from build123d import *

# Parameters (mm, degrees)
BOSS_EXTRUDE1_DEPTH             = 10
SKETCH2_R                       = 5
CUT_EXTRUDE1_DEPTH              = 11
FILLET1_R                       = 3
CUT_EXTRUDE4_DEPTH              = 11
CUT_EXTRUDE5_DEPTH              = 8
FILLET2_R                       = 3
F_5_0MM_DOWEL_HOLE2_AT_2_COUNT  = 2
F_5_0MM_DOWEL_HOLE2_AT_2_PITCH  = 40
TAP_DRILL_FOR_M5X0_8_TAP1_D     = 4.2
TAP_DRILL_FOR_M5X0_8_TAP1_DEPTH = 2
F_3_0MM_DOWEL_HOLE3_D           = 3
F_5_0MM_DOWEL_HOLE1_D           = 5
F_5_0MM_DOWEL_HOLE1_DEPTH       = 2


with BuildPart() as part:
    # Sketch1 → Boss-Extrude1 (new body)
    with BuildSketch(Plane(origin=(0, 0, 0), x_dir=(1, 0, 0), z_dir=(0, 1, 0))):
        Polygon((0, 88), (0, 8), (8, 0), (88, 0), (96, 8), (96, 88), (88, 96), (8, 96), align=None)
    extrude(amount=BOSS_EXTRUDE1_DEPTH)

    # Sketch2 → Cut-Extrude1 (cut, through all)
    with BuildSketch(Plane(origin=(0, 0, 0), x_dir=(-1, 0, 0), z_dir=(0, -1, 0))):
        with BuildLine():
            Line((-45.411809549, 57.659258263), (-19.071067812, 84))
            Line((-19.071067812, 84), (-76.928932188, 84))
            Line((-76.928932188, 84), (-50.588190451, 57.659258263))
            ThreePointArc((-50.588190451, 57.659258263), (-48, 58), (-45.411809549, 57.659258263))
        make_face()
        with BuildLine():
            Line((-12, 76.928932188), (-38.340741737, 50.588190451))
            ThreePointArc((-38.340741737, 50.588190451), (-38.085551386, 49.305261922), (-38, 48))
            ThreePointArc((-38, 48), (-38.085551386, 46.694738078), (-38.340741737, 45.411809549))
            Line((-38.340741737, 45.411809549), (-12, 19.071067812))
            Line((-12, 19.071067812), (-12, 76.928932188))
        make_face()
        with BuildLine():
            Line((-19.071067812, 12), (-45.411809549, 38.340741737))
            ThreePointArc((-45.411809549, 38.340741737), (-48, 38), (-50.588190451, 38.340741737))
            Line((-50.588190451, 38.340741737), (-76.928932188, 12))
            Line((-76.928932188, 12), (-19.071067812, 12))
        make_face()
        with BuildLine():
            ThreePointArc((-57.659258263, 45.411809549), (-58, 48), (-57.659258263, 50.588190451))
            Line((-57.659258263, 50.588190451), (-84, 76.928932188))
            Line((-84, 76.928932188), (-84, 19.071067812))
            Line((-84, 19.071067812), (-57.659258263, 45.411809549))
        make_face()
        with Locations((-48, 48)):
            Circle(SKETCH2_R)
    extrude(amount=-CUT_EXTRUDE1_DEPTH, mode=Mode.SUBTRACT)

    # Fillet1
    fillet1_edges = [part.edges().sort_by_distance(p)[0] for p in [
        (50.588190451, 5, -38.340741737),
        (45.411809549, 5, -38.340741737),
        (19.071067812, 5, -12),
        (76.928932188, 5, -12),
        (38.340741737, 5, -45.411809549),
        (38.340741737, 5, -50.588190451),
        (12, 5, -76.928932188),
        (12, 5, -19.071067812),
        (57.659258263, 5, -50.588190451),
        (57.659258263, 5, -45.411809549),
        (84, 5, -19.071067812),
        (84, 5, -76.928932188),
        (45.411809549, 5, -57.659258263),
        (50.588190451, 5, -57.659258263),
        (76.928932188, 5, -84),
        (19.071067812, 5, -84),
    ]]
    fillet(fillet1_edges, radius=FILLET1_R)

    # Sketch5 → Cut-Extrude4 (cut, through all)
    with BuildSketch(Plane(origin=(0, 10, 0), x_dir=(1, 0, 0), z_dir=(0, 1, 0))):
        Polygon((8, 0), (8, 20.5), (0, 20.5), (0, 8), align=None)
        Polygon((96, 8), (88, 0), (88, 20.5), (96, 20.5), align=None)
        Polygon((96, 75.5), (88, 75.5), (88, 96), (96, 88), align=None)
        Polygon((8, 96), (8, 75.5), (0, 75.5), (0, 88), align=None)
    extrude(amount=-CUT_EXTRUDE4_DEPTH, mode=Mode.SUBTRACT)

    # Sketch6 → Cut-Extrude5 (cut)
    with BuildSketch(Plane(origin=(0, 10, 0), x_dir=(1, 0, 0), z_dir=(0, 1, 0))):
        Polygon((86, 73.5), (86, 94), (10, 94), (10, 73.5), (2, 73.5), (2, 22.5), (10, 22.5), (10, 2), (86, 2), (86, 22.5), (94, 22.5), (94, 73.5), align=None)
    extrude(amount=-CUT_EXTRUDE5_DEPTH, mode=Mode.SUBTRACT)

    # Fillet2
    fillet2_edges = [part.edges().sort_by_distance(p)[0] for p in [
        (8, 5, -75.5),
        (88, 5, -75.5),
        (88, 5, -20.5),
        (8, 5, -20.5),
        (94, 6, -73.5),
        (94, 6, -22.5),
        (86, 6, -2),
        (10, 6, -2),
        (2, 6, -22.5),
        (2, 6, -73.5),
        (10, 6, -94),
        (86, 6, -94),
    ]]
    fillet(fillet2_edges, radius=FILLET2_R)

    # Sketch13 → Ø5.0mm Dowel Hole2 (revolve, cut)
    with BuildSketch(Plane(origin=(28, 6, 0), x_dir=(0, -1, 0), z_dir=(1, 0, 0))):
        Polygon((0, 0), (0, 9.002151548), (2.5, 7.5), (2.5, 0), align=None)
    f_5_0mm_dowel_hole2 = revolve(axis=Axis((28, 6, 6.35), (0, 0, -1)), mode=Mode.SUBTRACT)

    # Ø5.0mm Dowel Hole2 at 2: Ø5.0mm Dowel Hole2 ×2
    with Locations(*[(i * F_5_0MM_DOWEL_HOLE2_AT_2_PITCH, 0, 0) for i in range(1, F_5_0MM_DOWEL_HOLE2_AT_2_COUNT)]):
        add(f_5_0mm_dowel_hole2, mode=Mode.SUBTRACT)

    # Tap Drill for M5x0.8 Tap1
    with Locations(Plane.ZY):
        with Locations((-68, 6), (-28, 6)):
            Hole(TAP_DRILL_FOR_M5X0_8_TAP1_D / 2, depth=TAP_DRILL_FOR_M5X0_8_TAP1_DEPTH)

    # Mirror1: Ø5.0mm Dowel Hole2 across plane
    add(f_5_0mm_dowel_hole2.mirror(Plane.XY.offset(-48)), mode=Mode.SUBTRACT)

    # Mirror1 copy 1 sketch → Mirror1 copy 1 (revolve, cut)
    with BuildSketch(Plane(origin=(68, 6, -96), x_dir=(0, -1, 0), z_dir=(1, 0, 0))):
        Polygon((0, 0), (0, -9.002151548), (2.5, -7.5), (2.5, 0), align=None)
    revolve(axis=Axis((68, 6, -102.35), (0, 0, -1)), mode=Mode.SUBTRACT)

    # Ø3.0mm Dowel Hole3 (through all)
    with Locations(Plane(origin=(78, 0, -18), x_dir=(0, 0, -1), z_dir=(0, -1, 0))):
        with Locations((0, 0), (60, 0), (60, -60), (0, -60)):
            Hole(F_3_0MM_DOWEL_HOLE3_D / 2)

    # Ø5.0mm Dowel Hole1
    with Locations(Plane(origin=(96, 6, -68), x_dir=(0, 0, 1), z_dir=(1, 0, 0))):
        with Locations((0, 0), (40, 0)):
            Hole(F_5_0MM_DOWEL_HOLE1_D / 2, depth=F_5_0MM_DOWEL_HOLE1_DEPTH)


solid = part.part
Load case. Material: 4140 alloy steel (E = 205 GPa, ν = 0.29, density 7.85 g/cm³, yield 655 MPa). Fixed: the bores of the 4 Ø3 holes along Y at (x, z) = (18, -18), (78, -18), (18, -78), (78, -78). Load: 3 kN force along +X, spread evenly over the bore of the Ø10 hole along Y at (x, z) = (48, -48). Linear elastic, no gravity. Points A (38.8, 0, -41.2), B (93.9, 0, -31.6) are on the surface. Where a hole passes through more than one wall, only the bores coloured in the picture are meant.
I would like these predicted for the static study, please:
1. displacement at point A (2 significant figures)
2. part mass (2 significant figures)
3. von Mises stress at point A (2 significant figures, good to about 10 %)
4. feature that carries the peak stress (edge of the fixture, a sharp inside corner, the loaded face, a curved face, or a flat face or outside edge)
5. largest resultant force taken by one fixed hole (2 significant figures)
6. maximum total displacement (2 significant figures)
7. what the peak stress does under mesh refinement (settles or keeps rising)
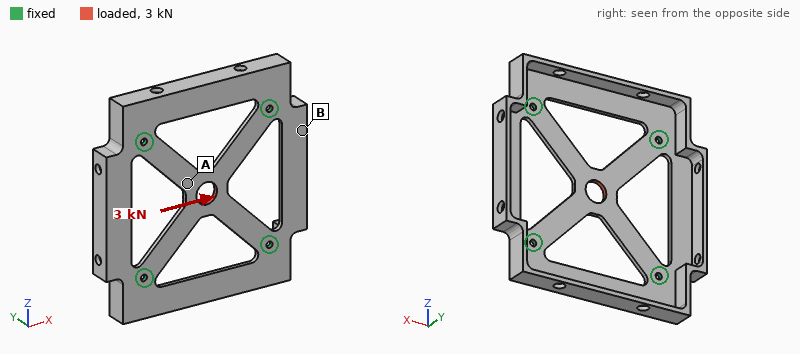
12 µm
130 g
44 MPa
edge of the fixture
980 N
15 µm
keeps rising
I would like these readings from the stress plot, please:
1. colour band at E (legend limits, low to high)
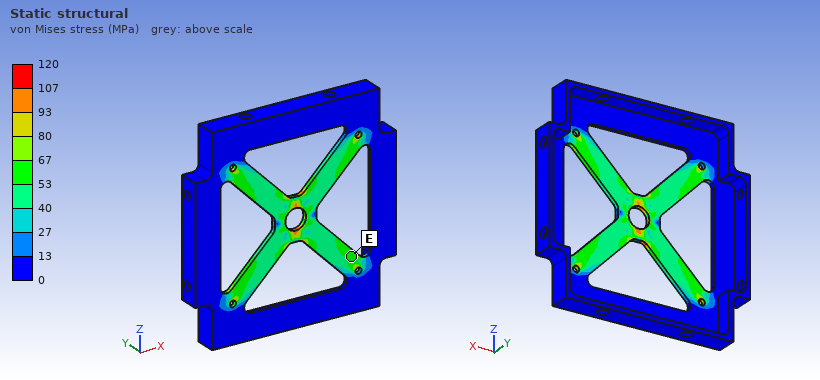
53 to 67 MPa
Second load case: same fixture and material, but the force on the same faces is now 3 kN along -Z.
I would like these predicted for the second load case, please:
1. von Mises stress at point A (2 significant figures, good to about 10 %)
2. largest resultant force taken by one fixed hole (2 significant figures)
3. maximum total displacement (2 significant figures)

46 MPa
980 N
15 µm
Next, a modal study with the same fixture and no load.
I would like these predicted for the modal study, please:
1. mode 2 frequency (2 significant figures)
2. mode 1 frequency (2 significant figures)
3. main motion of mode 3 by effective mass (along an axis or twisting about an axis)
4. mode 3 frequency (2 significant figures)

2300 Hz
1800 Hz
twisting about Z
2600 Hz
